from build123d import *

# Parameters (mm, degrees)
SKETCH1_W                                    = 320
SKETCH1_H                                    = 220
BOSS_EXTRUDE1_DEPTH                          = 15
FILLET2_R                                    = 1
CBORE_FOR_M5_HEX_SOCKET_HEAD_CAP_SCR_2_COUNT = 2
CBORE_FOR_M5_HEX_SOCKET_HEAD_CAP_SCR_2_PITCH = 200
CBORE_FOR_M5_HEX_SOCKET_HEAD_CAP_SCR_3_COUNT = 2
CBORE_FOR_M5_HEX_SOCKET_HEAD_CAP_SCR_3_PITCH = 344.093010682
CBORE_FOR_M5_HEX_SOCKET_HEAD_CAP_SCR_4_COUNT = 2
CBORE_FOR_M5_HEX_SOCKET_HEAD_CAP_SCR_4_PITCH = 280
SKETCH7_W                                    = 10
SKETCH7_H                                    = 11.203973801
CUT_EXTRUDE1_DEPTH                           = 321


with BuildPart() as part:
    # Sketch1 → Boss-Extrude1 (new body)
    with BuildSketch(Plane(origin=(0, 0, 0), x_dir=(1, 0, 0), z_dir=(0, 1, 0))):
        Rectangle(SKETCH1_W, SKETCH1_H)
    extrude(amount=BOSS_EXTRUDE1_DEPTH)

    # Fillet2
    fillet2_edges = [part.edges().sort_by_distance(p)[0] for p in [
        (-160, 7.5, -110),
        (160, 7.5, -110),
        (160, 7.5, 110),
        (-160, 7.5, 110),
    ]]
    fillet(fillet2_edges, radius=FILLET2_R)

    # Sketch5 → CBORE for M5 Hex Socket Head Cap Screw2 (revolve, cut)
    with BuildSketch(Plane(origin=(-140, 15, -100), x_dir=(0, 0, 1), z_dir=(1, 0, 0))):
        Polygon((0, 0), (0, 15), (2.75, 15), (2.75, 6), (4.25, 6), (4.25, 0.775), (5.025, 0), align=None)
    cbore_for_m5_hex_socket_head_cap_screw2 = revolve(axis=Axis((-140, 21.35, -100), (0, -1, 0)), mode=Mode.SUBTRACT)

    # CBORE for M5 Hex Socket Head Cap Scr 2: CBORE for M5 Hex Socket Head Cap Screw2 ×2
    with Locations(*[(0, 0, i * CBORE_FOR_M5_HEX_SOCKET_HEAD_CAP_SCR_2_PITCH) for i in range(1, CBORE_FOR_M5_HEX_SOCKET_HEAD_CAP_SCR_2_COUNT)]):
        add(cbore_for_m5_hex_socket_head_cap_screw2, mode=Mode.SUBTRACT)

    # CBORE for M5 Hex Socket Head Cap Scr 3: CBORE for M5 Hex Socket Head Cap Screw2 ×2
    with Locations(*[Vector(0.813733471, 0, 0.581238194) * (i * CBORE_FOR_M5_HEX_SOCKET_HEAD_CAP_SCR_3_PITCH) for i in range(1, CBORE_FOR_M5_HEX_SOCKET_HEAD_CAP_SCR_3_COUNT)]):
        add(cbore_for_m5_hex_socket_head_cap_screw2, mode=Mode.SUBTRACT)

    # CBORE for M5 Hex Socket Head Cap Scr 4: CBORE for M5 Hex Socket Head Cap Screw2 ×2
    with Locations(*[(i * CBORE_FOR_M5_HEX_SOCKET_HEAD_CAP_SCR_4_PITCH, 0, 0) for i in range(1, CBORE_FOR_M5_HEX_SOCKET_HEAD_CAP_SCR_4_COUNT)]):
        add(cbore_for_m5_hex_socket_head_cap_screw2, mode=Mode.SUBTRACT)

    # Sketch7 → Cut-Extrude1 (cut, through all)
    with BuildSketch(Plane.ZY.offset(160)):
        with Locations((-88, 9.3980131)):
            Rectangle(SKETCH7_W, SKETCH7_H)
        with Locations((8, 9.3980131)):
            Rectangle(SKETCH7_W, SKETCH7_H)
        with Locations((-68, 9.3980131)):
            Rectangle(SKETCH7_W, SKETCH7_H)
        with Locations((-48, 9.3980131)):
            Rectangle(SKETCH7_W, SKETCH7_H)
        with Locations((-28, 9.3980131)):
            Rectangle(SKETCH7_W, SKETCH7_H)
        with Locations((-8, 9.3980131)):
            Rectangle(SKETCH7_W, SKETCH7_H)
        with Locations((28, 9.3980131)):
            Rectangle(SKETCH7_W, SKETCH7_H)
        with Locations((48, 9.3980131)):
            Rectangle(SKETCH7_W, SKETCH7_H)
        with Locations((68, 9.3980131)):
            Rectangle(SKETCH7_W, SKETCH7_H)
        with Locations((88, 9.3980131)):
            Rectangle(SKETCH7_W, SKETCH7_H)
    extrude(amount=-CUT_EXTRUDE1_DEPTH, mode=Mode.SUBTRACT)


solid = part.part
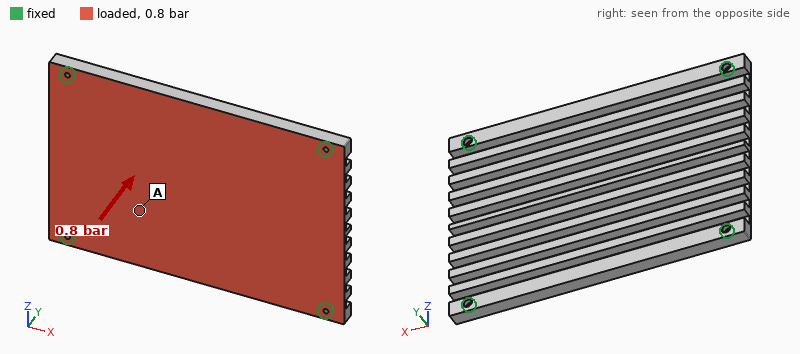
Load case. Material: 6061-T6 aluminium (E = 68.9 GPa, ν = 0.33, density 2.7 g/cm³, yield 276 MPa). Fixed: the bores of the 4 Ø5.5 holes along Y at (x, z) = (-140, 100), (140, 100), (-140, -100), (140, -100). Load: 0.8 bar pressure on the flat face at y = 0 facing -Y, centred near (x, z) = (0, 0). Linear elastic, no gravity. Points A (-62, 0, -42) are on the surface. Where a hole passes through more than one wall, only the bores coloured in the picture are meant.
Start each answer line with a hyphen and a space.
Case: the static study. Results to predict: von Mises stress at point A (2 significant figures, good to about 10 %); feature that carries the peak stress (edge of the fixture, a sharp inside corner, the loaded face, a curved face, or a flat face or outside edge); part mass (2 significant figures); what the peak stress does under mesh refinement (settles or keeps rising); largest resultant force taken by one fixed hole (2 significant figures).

- 16 MPa
- edge of the fixture
- 1.9 kg
- keeps rising
- 1.6 kN
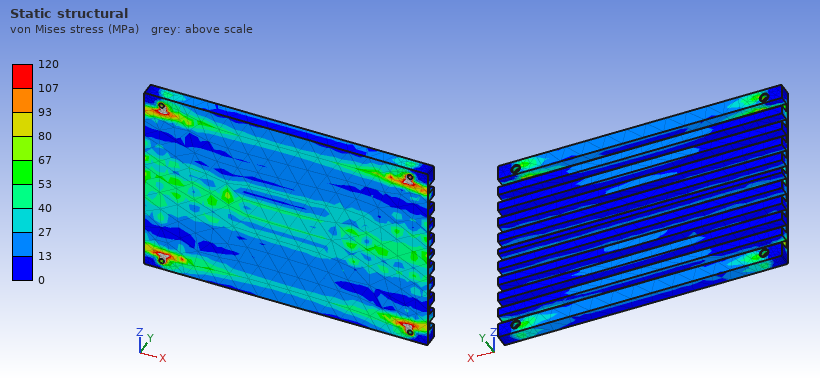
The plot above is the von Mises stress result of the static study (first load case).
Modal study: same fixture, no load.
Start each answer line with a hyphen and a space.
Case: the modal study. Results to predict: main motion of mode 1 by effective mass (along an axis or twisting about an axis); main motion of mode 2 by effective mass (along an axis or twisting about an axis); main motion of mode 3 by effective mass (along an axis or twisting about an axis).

- along Y
- twisting about Z
- twisting about X
